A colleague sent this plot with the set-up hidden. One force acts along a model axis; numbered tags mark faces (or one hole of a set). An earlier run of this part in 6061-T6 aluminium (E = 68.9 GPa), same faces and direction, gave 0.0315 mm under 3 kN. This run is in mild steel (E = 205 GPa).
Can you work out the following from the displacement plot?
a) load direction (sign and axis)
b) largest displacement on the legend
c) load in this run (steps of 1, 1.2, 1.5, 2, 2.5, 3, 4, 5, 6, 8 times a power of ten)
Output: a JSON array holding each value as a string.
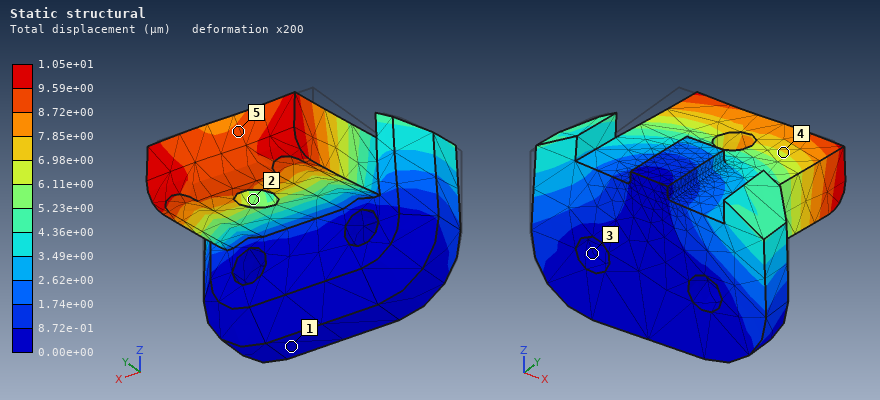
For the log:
["+X", "1.05e+01 µm", "3 kN"]
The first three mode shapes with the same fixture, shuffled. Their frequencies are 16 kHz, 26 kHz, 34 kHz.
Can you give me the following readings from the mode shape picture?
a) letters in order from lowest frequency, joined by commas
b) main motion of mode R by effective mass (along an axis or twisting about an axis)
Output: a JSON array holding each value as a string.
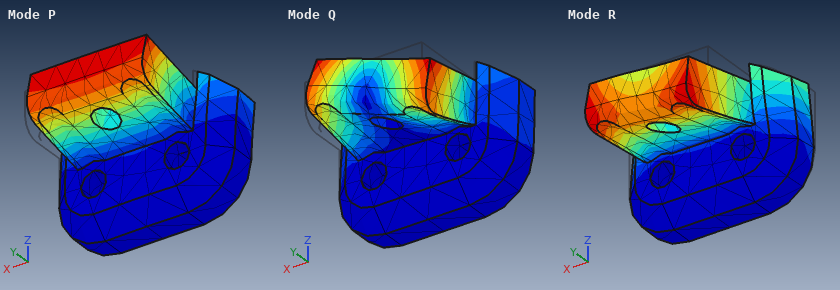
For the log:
["P, R, Q", "along X"]
